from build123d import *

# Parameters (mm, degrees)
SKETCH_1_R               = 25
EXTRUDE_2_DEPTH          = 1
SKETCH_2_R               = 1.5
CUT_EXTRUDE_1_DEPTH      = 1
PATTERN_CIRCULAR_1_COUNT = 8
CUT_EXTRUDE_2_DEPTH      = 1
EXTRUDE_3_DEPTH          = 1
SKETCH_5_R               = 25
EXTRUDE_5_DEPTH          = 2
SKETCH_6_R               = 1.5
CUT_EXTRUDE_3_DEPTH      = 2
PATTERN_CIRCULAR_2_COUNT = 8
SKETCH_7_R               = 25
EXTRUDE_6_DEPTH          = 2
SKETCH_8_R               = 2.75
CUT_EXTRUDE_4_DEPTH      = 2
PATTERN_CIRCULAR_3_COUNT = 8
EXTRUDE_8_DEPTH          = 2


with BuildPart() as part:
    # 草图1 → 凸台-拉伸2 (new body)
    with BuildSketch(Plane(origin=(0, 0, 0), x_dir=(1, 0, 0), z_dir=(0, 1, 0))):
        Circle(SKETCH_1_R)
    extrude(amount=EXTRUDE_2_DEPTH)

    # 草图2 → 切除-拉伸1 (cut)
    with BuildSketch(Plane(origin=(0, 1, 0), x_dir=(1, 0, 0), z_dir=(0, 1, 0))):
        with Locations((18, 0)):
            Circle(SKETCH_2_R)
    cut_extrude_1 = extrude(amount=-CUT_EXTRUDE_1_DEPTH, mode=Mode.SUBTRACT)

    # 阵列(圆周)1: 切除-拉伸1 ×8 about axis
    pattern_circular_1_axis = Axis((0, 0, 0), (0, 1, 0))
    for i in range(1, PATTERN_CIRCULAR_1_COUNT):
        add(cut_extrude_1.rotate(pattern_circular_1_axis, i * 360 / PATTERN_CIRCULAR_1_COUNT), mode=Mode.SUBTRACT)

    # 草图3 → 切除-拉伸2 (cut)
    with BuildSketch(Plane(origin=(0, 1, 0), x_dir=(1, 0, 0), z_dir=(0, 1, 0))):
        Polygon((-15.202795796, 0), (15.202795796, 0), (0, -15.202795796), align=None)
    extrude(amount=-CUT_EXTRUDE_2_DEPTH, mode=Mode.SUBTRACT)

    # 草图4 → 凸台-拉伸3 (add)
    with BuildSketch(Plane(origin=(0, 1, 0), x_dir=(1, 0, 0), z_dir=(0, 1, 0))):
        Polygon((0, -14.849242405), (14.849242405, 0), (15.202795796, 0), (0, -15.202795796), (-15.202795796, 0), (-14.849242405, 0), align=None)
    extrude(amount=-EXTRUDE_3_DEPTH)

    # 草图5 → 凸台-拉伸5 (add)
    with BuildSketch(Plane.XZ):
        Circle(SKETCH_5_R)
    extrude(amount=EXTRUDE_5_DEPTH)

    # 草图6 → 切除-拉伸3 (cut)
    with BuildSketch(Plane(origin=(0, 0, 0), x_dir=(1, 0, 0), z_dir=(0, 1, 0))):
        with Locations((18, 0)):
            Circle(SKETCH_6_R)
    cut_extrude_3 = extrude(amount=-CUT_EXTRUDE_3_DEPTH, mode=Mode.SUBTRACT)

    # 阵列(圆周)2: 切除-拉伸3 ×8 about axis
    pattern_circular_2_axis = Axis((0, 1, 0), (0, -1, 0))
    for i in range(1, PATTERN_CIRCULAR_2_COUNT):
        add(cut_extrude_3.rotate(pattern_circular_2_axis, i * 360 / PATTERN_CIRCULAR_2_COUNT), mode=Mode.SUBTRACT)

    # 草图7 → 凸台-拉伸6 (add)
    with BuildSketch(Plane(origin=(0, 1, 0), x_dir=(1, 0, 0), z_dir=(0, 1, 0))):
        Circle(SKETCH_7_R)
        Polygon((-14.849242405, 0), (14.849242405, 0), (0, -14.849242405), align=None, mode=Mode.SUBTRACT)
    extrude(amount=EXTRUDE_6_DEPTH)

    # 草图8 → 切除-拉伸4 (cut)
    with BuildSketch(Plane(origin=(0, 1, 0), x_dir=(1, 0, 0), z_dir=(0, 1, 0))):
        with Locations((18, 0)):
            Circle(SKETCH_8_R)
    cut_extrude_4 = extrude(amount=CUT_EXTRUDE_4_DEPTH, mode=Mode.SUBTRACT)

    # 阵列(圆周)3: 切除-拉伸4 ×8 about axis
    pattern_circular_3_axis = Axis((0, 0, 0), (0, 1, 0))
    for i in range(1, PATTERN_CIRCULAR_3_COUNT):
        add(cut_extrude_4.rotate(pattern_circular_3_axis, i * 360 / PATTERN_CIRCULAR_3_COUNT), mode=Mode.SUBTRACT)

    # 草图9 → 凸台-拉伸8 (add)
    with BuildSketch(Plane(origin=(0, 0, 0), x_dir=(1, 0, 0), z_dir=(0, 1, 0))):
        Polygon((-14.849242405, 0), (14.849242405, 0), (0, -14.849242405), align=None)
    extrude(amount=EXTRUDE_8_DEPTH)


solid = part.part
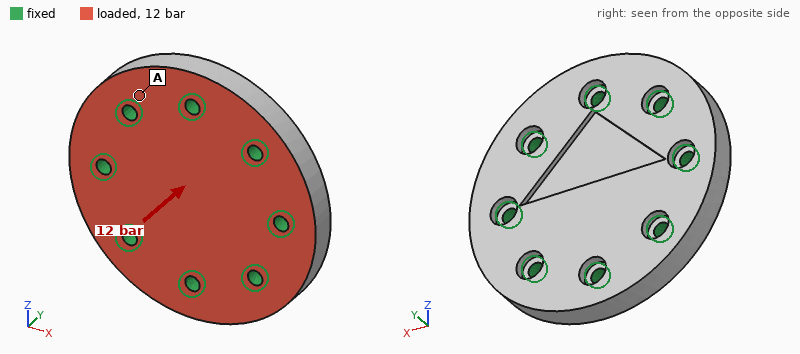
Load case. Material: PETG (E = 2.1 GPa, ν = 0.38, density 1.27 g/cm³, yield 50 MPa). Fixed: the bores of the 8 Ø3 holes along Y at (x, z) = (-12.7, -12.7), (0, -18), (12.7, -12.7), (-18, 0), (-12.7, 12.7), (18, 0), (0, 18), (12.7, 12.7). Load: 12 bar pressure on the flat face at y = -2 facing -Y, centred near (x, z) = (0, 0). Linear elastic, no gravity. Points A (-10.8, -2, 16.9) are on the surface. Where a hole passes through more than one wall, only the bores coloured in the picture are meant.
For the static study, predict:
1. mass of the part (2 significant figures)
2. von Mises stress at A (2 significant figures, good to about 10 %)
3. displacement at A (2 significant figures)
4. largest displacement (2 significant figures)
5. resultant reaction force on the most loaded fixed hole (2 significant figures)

11 g
4.6 MPa
0.024 mm
0.15 mm
290 N
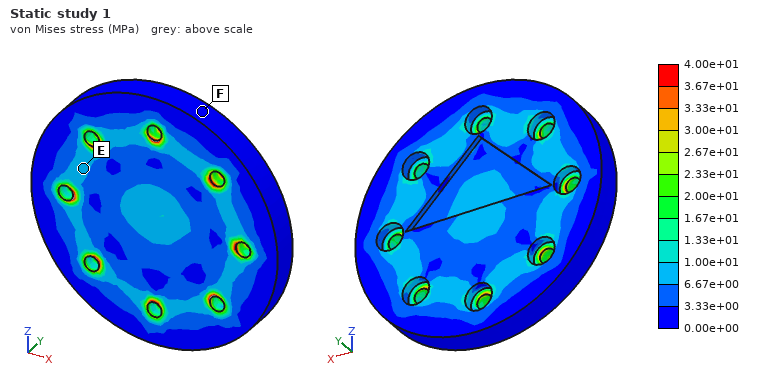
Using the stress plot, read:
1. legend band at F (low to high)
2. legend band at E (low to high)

0.00e+00 to 3.33e+00 MPa
6.67e+00 to 1.00e+01 MPa
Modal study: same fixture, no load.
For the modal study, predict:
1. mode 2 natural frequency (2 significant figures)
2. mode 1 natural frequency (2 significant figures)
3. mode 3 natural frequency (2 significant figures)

9700 Hz
6300 Hz
9700 Hz
